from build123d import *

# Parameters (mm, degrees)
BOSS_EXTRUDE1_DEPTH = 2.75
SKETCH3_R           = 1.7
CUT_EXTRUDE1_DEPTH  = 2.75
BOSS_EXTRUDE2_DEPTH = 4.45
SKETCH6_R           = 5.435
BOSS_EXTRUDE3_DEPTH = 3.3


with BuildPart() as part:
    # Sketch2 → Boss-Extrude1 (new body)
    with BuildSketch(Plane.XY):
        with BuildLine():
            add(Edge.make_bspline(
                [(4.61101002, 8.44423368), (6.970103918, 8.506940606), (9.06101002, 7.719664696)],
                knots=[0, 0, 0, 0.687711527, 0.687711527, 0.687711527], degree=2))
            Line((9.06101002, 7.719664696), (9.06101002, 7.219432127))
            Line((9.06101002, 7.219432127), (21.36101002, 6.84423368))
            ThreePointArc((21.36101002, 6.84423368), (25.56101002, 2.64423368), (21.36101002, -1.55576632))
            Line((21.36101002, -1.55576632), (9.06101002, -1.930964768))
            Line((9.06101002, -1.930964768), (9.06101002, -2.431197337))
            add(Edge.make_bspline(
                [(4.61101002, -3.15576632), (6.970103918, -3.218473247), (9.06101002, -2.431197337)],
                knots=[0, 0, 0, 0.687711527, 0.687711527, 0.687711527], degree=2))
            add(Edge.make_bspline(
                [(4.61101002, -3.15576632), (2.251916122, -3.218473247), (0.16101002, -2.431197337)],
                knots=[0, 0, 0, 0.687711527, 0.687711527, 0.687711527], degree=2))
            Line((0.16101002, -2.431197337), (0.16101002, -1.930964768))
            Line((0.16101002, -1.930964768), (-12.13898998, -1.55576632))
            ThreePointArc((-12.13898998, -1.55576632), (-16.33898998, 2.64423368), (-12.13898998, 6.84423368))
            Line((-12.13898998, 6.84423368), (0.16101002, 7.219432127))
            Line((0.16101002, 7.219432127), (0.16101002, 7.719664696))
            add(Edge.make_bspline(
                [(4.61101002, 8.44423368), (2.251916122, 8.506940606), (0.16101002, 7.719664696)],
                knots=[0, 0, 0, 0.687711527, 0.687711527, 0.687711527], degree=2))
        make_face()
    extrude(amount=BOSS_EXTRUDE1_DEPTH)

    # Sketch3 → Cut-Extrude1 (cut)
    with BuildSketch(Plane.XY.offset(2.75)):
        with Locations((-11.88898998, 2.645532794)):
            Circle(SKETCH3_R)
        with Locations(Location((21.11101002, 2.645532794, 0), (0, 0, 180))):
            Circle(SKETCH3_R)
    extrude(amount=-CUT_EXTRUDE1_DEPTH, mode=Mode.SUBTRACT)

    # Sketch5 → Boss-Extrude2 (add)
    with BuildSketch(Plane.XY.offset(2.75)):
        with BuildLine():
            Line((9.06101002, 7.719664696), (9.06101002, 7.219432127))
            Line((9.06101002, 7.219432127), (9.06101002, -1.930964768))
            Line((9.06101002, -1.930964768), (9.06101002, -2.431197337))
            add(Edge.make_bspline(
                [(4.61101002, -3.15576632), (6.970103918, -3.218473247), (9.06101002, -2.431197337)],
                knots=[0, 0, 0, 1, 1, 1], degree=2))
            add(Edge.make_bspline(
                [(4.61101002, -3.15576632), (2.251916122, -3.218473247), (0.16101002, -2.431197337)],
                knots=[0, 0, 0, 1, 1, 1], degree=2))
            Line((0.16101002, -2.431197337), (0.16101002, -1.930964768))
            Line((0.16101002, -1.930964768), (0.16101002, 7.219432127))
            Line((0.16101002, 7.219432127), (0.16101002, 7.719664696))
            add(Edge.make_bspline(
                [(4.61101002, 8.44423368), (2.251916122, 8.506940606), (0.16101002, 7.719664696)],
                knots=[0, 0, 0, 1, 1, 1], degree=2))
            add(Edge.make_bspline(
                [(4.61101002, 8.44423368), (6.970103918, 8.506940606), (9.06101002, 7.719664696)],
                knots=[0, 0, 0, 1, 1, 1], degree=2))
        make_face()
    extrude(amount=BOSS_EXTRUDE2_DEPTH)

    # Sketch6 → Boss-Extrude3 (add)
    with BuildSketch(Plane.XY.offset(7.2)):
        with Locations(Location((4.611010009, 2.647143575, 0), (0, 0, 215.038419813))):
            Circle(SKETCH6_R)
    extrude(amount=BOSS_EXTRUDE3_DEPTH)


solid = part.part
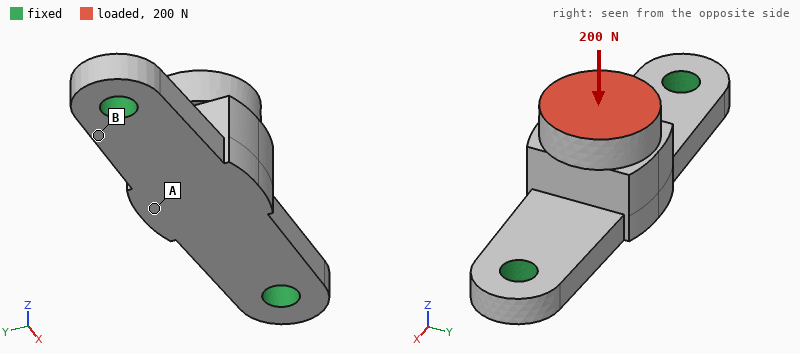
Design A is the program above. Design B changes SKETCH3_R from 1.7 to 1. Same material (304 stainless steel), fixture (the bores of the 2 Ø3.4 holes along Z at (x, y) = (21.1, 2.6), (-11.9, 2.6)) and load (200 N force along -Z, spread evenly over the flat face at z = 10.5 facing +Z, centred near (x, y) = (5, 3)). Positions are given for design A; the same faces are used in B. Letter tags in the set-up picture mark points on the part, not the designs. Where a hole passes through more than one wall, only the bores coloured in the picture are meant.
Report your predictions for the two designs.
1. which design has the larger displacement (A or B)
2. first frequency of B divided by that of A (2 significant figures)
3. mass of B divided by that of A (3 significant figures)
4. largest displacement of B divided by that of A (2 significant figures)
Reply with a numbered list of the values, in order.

1. B
2. 0.93
3. 1.02
4. 1.2
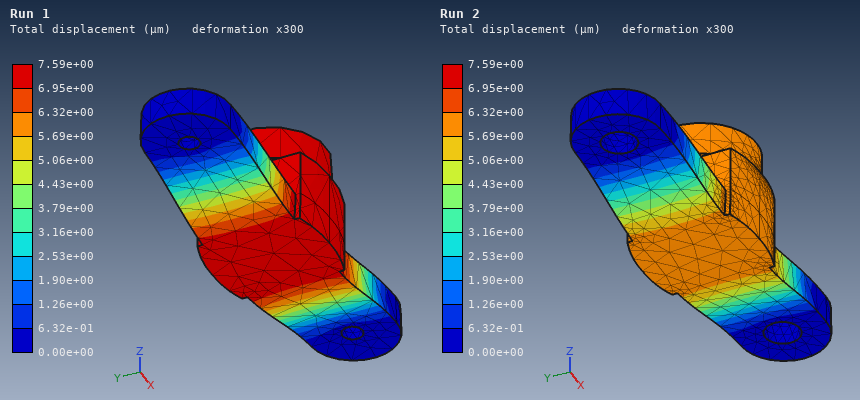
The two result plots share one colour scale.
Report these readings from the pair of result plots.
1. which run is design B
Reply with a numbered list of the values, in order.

1. Run 1
